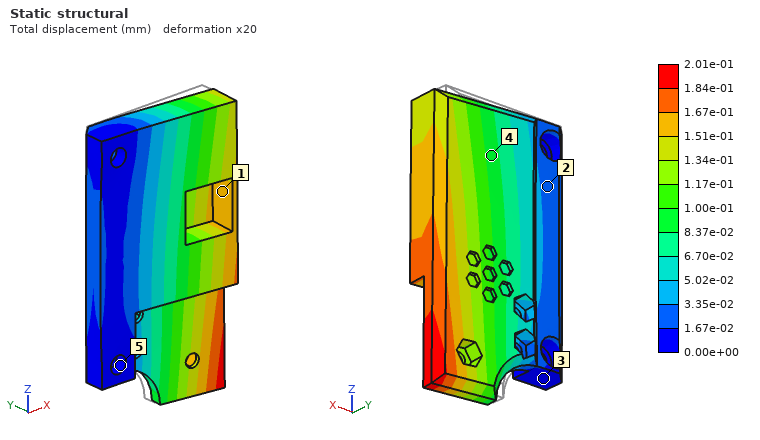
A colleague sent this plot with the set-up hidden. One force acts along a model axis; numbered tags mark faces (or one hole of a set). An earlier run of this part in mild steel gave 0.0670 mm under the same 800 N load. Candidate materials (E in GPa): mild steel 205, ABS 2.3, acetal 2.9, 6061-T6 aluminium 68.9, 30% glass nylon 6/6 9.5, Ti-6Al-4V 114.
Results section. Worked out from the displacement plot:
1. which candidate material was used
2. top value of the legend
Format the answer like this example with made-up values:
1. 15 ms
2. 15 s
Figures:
1. 6061-T6 aluminium
2. 2.01e-01 mm
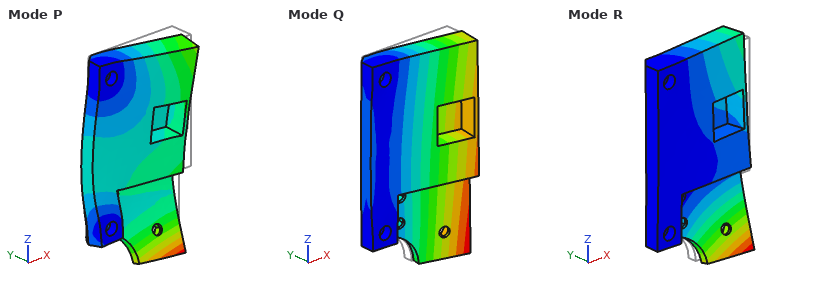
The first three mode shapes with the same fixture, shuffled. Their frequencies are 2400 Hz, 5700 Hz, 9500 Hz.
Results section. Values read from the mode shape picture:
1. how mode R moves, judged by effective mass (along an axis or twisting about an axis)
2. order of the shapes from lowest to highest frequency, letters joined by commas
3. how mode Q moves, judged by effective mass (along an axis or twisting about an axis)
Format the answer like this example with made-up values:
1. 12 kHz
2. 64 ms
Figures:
1. twisting about X
2. Q, R, P
3. along Y
